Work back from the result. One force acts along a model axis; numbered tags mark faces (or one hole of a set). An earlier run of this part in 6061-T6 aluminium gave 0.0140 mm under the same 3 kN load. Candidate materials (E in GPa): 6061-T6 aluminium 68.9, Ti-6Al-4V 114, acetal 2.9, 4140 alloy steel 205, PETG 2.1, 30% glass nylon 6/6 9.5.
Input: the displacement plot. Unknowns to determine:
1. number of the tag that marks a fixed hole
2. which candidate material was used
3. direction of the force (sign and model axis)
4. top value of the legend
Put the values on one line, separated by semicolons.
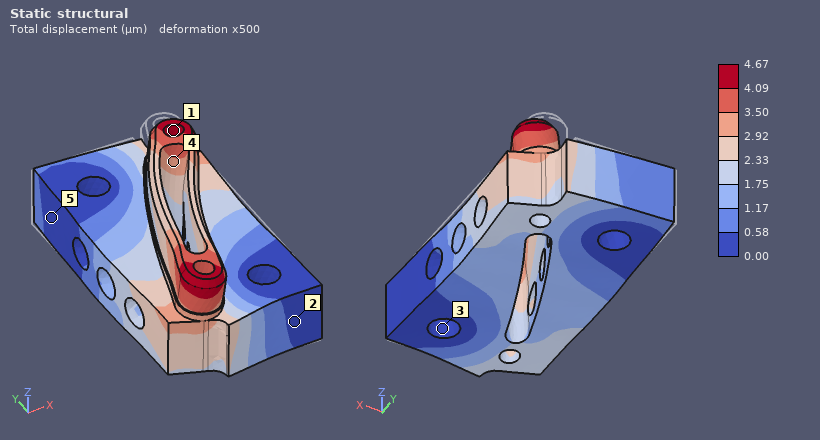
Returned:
3; 4140 alloy steel; -Y; 4.67 µm
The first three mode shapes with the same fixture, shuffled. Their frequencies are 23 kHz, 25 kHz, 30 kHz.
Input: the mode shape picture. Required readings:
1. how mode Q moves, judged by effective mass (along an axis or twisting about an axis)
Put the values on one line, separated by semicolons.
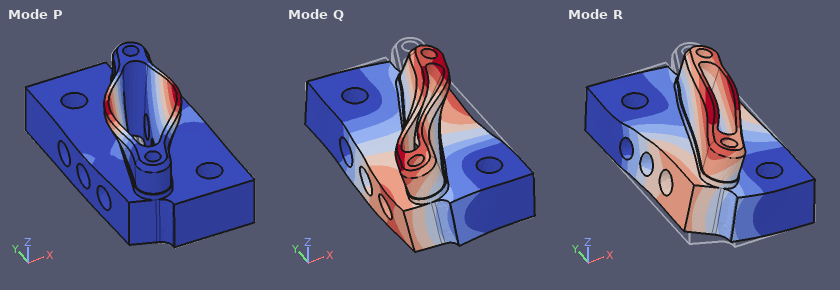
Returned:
along Z
